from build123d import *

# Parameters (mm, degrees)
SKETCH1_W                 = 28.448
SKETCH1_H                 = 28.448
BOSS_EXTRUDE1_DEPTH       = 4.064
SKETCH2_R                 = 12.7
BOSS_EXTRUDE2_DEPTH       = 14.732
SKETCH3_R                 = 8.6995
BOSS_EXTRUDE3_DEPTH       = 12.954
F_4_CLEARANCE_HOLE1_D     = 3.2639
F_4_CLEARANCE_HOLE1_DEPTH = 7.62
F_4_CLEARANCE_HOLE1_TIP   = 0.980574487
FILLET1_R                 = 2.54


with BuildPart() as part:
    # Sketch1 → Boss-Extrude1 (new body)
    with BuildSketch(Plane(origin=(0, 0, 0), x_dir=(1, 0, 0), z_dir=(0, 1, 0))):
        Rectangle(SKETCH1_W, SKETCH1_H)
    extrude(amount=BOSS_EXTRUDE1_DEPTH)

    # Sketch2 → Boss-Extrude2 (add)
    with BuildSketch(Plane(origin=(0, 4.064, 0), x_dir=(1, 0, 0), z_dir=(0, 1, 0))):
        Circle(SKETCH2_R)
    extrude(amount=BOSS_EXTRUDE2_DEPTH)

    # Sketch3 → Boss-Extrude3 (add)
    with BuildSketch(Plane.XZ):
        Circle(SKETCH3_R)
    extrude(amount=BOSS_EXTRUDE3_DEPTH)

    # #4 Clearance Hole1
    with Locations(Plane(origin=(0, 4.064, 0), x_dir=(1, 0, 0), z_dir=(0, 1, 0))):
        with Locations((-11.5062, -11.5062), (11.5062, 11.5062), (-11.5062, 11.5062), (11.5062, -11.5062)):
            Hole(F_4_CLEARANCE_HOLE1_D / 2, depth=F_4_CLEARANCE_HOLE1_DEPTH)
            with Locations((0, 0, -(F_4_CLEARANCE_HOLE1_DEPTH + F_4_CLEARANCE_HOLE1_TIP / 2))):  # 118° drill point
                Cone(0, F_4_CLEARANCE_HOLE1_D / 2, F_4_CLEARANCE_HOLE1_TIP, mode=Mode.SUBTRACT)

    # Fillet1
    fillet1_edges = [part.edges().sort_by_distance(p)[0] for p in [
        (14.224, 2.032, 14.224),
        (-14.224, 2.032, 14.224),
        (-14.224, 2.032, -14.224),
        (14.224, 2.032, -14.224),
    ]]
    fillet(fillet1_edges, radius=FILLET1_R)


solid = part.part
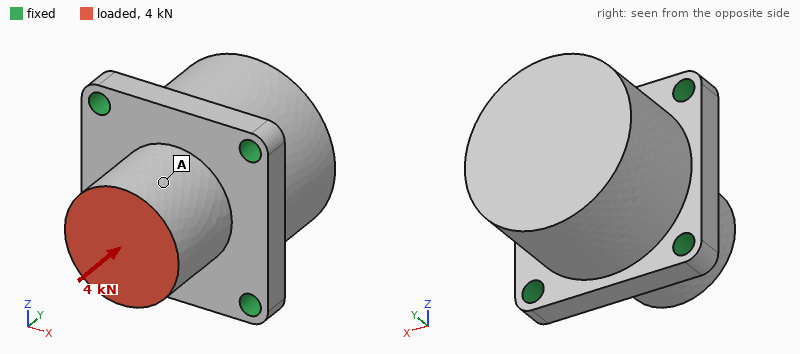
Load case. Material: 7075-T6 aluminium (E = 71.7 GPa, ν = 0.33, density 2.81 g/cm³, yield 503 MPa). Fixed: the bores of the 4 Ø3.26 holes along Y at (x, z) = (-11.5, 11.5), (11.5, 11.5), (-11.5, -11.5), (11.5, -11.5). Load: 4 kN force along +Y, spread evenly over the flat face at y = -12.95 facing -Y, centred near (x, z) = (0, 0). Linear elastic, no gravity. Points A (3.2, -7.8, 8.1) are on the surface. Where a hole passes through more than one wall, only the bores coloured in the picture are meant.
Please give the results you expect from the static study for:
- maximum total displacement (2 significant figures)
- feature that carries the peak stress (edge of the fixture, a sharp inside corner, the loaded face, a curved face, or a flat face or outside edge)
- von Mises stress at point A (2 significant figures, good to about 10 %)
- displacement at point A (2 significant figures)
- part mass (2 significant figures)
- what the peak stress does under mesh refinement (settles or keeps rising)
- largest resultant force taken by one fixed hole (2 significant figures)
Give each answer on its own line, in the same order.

13 µm
edge of the fixture
16 MPa
11 µm
38 g
keeps rising
1.0 kN
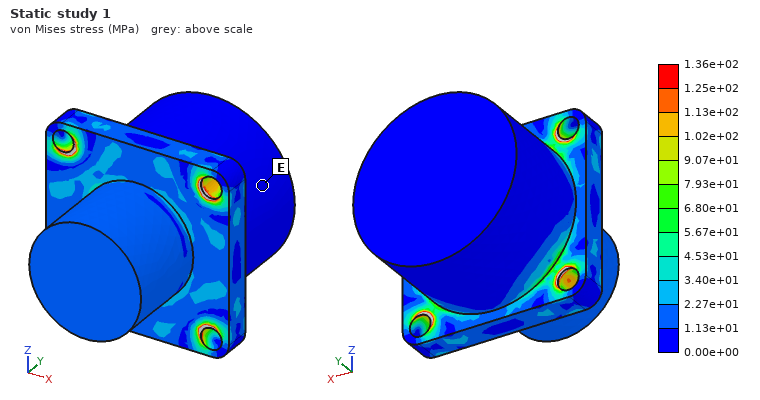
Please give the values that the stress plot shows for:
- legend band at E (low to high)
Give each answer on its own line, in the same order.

0.00e+00 to 1.13e+01 MPa
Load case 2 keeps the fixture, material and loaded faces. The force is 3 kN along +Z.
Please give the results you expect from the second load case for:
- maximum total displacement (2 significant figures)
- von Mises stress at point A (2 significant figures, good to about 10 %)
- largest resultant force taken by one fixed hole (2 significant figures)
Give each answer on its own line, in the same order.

44 µm
31 MPa
1.3 kN
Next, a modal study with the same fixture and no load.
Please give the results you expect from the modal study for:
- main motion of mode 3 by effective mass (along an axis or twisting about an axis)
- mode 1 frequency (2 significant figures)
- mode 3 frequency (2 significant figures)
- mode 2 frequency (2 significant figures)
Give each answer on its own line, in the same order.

along Y
16 kHz
18 kHz
16 kHz
